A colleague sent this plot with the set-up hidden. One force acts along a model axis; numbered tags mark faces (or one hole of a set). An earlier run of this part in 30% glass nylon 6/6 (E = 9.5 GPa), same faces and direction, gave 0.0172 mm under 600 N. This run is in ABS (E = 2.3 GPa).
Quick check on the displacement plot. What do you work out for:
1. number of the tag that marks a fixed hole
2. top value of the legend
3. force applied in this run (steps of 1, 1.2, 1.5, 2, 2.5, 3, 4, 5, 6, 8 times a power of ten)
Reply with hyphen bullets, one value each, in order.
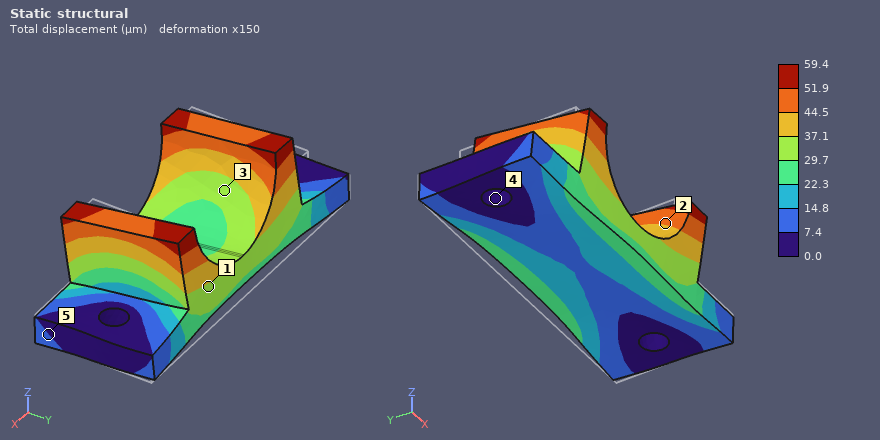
- 4
- 59.4 µm
- 500 N
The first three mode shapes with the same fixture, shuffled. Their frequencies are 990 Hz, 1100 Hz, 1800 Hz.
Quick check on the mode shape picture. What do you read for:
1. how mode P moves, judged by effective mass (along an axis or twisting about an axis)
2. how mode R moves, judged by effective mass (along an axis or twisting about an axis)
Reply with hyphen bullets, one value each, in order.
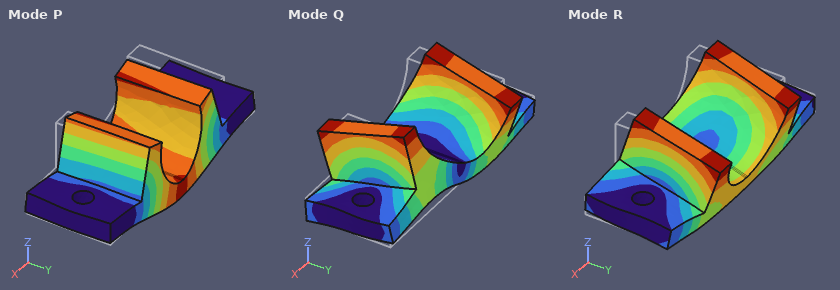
- along Z
- along Y
